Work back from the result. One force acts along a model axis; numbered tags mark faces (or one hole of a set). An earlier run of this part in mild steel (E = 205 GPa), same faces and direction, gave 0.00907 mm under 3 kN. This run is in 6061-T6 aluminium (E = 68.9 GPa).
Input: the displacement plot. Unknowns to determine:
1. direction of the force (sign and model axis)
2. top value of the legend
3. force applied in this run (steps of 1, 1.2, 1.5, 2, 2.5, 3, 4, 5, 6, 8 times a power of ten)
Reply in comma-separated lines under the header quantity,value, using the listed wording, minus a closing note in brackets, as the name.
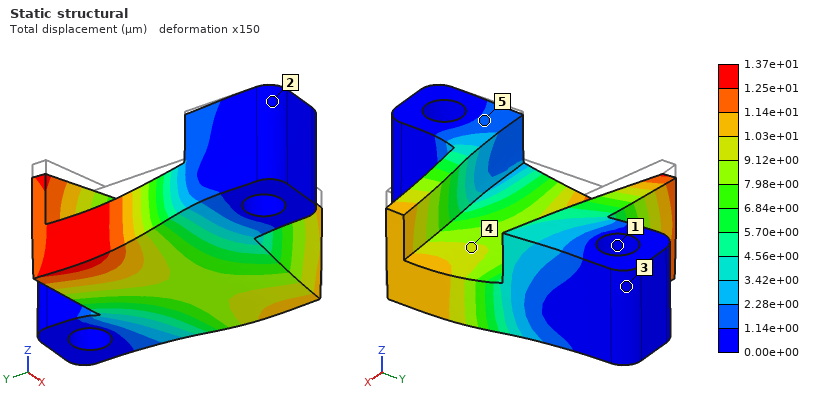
quantity,value
direction of the force,-Z
top value of the legend,1.37e+01 µm
force applied in this run,1.5 kN
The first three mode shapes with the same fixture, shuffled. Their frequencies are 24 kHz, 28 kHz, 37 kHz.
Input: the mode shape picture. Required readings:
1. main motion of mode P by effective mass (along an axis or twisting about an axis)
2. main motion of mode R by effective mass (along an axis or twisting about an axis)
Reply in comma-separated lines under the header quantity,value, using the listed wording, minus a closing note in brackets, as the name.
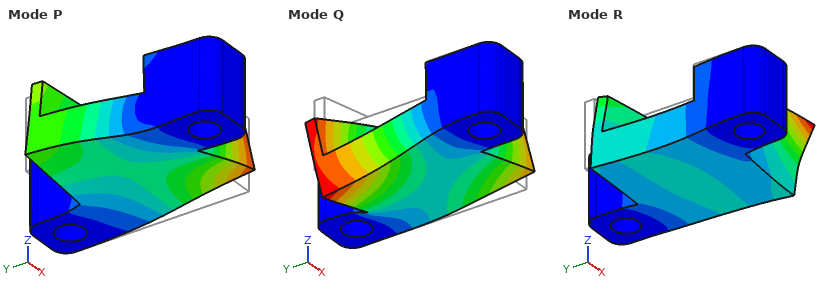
quantity,value
main motion of mode P by effective mass,along Z
main motion of mode R by effective mass,along X
